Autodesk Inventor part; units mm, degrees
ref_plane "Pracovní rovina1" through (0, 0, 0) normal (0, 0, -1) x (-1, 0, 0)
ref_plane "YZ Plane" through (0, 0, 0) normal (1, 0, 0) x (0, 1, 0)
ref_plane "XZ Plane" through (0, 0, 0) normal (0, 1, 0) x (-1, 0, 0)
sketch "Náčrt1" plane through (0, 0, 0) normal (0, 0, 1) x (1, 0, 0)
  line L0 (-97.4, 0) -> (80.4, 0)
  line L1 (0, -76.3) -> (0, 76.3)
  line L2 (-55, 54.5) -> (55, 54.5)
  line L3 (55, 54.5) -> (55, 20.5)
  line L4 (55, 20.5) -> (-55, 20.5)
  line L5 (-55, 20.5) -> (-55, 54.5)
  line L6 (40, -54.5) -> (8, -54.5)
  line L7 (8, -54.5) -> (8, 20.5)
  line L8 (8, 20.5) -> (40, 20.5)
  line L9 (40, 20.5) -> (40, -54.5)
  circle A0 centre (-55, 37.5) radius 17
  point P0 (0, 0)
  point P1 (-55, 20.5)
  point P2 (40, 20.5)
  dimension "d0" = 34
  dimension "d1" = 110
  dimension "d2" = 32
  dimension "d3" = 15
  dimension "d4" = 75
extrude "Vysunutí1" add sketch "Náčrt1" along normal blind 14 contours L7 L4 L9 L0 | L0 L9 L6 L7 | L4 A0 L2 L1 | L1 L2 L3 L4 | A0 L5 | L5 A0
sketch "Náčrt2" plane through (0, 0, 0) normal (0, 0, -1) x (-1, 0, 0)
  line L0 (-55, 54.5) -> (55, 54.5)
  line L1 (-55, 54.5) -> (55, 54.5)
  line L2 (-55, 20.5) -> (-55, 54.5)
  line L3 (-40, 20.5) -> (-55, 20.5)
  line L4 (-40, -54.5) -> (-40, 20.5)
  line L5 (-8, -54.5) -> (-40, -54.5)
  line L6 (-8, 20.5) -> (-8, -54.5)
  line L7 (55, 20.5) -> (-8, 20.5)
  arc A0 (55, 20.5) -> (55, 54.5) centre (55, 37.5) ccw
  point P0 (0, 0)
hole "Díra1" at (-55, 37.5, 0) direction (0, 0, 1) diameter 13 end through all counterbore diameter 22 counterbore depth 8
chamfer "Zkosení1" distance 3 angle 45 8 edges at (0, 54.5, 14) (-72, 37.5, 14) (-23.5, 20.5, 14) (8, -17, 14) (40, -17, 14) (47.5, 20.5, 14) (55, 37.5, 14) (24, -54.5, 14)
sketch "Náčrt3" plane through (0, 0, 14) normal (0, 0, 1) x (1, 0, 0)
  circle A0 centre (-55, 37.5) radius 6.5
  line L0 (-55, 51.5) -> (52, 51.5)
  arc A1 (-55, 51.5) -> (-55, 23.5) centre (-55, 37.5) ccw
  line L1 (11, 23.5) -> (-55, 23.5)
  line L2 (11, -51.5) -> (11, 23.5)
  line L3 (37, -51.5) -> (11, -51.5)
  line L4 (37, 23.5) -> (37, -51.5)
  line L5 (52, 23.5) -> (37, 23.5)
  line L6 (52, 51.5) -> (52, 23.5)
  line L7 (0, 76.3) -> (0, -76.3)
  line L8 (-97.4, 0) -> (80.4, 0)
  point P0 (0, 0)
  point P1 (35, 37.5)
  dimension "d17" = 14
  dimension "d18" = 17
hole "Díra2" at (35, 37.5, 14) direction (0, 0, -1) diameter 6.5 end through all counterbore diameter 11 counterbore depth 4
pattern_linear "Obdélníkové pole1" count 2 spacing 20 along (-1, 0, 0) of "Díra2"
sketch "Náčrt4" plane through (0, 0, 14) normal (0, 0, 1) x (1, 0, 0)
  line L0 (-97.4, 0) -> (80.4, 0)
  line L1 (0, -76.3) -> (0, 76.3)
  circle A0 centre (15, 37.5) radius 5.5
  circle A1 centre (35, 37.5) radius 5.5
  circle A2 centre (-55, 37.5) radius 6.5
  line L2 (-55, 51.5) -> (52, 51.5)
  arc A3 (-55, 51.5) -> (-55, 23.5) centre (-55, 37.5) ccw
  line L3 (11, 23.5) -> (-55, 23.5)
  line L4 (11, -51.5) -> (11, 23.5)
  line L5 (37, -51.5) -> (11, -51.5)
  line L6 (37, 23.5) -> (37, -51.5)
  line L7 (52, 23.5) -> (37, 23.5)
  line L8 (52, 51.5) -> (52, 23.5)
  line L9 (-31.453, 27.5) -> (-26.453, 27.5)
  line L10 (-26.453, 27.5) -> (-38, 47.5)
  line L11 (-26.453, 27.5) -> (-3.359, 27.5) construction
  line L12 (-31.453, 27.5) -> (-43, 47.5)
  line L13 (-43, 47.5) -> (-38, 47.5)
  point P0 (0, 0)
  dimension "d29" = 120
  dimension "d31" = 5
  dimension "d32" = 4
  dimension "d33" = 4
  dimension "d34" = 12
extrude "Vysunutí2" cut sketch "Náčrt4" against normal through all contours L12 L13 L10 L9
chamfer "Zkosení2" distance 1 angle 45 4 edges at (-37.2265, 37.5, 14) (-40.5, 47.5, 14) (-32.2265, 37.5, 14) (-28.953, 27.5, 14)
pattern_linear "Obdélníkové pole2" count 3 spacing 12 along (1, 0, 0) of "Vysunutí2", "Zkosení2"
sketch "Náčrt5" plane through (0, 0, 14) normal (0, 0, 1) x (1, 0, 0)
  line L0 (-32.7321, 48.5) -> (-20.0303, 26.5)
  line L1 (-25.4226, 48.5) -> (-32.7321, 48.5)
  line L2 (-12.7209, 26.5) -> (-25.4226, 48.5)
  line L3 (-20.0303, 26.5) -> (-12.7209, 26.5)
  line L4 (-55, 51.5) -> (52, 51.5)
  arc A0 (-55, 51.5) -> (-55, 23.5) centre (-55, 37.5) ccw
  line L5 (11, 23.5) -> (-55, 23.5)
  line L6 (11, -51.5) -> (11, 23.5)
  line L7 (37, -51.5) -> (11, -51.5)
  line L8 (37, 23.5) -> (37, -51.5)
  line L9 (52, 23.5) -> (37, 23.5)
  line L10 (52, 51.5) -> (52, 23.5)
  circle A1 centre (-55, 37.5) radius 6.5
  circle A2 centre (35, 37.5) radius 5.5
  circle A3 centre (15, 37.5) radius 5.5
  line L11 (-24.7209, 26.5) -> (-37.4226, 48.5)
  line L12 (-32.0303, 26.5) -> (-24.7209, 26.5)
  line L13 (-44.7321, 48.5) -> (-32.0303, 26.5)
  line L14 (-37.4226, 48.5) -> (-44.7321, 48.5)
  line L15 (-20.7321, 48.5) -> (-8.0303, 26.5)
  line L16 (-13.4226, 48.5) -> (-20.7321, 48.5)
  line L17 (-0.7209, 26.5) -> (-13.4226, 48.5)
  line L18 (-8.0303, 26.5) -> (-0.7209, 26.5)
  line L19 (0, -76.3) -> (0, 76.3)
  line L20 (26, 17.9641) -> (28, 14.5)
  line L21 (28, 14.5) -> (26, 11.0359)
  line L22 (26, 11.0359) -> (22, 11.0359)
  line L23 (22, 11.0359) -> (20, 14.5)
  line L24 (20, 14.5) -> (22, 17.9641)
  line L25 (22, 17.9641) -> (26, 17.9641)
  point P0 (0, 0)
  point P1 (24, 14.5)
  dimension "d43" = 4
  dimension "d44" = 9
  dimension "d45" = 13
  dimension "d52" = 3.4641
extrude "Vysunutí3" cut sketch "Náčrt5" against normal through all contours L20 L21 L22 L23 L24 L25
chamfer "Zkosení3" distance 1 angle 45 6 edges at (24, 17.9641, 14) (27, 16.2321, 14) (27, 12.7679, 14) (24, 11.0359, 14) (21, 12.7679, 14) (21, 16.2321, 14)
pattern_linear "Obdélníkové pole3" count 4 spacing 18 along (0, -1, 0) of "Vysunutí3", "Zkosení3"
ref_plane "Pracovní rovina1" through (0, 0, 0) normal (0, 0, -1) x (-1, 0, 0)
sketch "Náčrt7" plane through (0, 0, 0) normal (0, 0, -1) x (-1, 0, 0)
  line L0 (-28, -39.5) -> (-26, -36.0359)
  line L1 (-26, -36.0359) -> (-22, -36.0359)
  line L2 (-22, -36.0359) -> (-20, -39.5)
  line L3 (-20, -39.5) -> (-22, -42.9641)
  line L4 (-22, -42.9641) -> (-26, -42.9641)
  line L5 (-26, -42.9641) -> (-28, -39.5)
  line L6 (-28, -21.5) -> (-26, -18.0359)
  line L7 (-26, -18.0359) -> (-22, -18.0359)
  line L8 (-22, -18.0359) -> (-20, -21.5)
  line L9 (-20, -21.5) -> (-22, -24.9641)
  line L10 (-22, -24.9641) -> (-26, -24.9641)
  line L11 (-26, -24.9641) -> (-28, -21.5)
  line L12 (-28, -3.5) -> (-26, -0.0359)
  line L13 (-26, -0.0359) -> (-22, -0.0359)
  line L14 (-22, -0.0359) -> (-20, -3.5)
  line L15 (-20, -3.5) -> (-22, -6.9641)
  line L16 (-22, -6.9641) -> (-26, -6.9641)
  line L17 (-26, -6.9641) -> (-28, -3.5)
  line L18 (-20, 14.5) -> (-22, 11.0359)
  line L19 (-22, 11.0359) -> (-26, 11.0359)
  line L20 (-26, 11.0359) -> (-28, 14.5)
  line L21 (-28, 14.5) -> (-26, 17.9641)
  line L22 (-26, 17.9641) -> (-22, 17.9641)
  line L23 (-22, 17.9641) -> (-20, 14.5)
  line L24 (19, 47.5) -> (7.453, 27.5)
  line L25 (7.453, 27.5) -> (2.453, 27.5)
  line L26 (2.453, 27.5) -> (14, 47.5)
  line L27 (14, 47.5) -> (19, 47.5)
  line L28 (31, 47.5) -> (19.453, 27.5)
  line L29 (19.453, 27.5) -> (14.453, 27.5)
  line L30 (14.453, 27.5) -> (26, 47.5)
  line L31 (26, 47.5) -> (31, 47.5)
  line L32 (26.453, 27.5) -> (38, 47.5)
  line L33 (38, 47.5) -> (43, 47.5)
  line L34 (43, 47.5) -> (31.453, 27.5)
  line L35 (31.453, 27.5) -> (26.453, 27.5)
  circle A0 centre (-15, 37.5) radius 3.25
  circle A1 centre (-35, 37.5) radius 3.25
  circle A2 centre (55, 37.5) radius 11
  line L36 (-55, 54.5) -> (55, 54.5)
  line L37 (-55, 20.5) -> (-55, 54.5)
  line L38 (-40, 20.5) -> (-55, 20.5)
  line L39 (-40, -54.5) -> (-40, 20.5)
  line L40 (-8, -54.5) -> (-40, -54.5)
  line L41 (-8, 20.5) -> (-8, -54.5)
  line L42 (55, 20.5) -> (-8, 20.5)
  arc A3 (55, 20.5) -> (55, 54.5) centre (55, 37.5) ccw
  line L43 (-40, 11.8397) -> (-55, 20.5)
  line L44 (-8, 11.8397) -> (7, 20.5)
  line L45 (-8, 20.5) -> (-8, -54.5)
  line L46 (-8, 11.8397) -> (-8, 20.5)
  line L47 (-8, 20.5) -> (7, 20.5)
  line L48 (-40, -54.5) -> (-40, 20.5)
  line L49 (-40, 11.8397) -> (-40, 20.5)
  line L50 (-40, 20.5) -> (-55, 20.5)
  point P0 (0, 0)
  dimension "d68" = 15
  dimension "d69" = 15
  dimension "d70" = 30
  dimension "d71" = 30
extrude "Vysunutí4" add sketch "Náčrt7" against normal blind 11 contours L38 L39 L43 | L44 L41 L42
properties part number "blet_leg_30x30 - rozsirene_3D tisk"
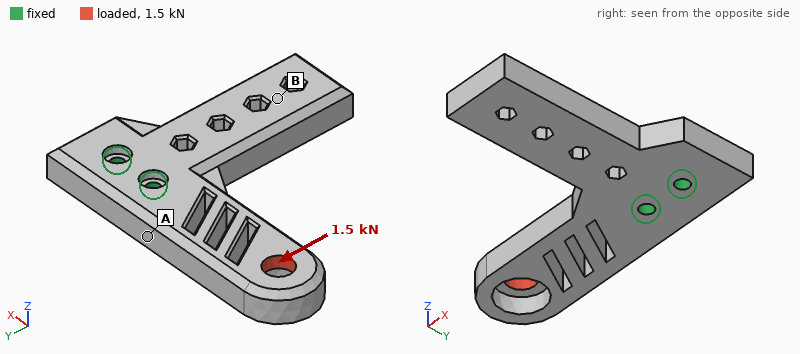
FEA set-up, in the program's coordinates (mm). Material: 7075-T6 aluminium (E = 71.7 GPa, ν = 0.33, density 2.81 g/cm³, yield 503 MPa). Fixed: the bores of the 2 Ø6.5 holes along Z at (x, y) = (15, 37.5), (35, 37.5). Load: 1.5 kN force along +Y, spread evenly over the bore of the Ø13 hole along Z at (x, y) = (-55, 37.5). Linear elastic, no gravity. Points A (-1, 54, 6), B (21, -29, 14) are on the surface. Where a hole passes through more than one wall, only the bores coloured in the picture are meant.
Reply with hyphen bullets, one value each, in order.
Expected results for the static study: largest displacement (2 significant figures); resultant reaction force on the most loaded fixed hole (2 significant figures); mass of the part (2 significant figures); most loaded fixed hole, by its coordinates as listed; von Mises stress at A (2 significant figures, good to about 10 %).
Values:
- 0.17 mm
- 5.3 kN
- 220 g
- (15, 37.5)
- 36 MPa
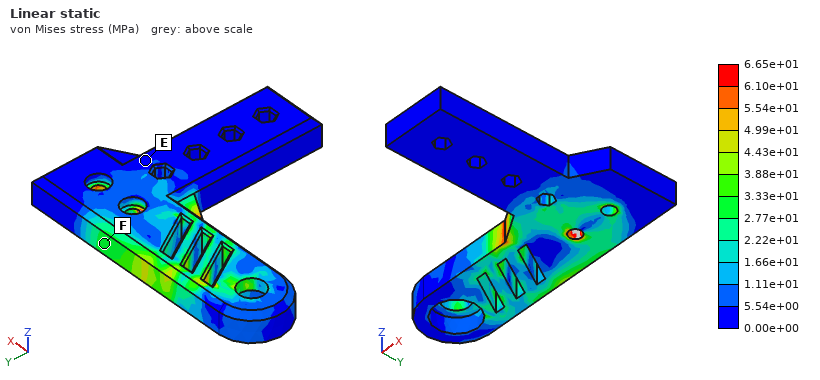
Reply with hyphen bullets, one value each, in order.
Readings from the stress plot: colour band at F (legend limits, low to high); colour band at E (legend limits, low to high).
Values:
- 2.77e+01 to 3.33e+01 MPa
- 0.00e+00 to 5.54e+00 MPa
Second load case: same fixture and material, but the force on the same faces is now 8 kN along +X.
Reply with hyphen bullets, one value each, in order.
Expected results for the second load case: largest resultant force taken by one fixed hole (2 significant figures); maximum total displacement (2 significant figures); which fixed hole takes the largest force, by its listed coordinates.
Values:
- 5.4 kN
- 0.46 mm
- (15, 37.5)
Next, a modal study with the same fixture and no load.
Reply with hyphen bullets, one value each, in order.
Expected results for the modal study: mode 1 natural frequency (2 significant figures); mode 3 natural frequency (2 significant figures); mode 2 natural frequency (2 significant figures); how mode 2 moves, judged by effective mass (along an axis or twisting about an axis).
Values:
- 1300 Hz
- 2700 Hz
- 1500 Hz
- along Z
